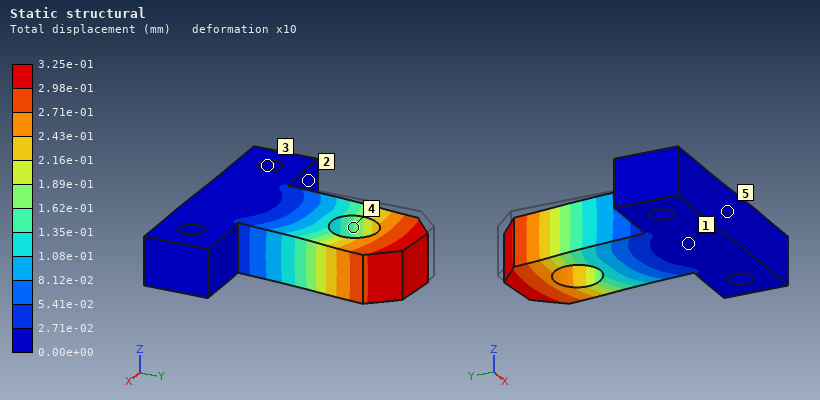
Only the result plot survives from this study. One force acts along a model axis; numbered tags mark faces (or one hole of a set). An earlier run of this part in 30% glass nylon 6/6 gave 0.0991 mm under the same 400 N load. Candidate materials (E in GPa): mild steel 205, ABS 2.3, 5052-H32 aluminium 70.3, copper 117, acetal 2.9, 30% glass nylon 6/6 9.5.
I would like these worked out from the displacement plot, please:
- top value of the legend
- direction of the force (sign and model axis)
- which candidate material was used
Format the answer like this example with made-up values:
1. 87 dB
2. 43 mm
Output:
1. 3.25e-01 mm
2. +X
3. acetal
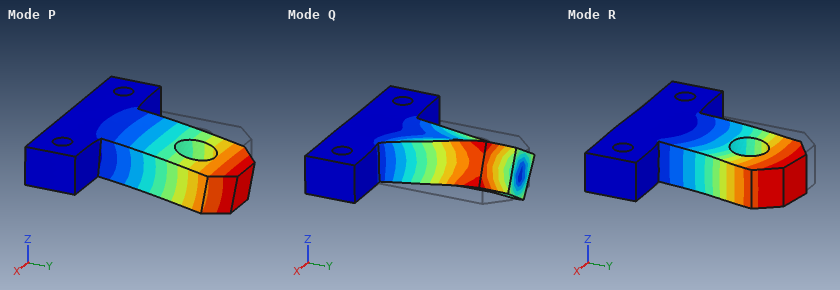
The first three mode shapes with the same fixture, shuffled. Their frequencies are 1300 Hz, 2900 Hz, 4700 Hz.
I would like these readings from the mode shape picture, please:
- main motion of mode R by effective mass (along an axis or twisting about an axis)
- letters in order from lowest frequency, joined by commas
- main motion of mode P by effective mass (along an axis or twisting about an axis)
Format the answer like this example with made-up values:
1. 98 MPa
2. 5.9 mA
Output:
1. along X
2. P, R, Q
3. along Z
